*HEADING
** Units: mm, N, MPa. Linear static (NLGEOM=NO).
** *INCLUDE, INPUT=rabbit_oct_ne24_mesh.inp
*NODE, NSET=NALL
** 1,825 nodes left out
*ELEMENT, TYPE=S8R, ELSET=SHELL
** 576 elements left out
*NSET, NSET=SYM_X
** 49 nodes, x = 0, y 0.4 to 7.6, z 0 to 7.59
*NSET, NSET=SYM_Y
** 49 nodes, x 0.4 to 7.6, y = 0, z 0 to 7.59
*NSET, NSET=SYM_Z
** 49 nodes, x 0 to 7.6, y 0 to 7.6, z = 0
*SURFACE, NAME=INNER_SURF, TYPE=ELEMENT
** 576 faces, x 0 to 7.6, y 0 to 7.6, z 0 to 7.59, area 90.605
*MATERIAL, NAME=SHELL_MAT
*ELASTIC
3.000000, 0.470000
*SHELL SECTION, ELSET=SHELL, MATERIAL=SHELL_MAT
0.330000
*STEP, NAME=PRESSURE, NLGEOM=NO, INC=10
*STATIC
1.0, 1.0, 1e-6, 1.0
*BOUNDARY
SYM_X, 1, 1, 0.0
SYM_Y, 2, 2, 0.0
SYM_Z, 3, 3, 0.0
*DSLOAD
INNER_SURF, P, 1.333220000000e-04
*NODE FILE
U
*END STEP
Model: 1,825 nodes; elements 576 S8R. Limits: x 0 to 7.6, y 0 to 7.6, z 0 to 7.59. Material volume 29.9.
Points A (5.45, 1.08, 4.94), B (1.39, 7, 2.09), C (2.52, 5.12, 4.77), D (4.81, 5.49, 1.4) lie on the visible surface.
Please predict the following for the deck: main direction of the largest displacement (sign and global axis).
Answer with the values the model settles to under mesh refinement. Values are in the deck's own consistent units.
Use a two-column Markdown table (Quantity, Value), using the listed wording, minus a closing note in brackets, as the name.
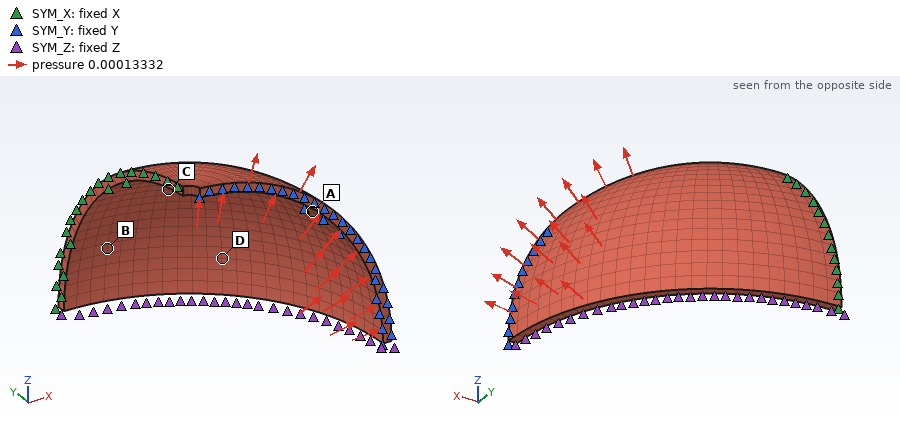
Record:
| Quantity | Value |
|---|---|
| main direction of the largest displacement | +X |
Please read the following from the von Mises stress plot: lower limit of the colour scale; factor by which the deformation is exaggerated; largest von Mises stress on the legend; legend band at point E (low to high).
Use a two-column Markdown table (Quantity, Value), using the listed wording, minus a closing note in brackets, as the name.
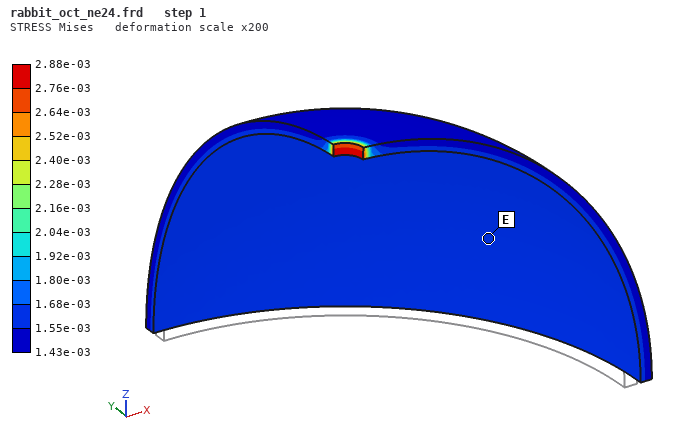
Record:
| Quantity | Value |
|---|---|
| lower limit of the colour scale | 1.43e-03 |
| factor by which the deformation is exaggerated | 200 |
| largest von Mises stress on the legend | 2.88e-03 |
| legend band at point E | 1.55e-03 to 1.68e-03 |
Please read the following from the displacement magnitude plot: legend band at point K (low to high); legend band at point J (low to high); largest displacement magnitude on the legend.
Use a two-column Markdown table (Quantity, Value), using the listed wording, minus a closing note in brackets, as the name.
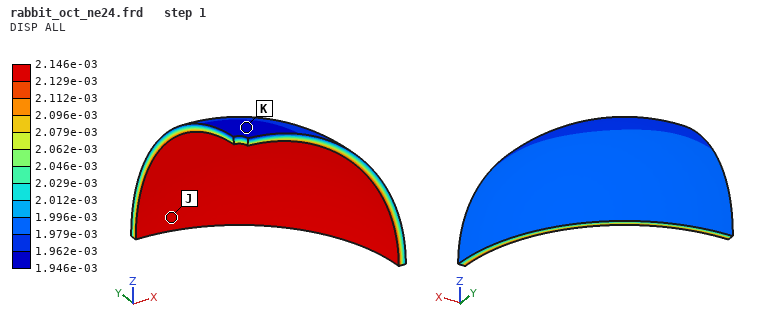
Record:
| Quantity | Value |
|---|---|
| legend band at point K | 1.946e-03 to 1.962e-03 |
| legend band at point J | 2.129e-03 to 2.146e-03 |
| largest displacement magnitude on the legend | 2.146e-03 |
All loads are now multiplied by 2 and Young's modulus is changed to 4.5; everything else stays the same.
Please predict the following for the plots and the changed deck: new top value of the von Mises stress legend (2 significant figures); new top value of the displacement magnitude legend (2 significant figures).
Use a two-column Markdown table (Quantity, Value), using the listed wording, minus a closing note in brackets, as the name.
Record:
| Quantity | Value |
|---|---|
| new top value of the von Mises stress legend | 0.0058 |
| new top value of the displacement magnitude legend | 0.0029 |
